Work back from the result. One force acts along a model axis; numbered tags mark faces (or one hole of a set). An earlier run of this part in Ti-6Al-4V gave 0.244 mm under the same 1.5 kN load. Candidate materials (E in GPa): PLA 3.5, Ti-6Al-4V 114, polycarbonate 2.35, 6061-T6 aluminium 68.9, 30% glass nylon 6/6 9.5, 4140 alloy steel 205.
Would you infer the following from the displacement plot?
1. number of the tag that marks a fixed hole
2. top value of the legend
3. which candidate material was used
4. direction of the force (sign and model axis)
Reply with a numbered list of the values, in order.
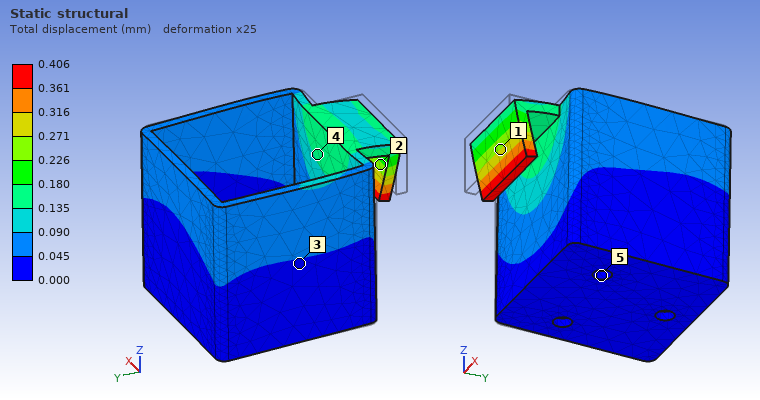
1. 5
2. 0.406 mm
3. 6061-T6 aluminium
4. +Y
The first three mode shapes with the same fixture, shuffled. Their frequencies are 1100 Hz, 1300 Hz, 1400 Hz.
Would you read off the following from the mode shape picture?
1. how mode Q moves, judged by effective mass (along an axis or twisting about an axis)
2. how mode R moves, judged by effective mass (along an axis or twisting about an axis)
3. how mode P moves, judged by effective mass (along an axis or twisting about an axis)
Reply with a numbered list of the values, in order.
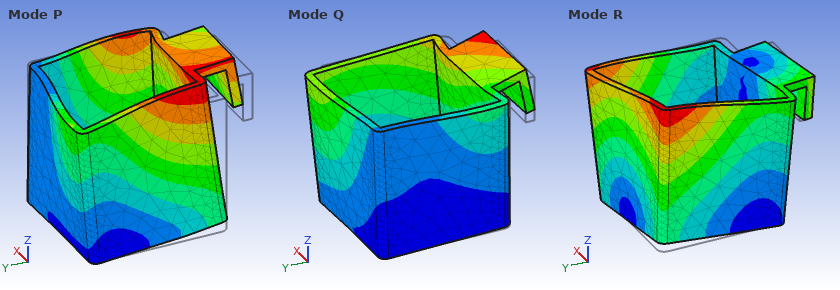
1. along Y
2. along X
3. along X
